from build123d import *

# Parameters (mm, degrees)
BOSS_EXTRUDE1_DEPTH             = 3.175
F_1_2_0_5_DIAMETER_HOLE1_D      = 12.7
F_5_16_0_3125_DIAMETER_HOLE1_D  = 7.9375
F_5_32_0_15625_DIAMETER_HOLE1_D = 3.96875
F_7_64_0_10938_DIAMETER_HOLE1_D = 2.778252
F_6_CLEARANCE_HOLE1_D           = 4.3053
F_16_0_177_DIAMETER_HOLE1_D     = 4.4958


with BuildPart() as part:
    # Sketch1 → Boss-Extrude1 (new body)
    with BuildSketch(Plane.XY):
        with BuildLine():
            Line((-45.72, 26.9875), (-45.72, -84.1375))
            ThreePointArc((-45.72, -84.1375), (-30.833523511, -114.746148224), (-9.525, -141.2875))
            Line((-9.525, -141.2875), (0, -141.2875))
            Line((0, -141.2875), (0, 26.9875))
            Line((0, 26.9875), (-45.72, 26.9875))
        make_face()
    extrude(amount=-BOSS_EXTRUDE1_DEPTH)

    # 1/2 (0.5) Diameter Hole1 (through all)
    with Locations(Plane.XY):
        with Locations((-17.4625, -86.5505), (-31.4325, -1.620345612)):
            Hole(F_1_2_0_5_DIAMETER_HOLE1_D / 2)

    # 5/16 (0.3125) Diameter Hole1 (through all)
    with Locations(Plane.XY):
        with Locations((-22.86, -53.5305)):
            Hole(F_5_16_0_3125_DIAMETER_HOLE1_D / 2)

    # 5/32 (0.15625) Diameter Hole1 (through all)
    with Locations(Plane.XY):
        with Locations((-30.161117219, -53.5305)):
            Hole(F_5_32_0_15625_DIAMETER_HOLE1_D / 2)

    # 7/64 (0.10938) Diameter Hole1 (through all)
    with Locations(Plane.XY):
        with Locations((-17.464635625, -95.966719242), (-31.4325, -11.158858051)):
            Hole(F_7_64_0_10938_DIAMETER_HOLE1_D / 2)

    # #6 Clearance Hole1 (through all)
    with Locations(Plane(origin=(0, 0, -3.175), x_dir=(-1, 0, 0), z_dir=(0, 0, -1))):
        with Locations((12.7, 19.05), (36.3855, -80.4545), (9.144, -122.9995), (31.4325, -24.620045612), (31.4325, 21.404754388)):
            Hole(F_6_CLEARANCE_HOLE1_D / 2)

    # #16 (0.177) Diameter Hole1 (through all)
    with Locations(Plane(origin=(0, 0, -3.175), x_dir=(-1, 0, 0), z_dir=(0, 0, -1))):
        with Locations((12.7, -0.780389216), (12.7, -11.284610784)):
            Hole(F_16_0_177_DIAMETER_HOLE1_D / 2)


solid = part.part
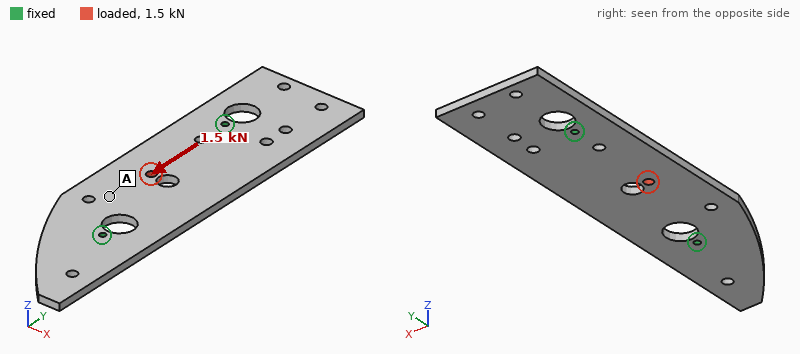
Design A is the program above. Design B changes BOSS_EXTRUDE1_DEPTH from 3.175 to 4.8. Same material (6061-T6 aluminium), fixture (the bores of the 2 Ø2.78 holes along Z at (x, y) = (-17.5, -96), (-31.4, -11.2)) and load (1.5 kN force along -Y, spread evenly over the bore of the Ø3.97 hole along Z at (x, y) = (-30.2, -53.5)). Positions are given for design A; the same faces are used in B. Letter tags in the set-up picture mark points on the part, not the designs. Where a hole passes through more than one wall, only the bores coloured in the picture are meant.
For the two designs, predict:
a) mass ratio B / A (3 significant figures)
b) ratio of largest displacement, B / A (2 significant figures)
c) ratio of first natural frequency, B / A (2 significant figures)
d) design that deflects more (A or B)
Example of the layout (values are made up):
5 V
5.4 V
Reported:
1.51
0.66
1.4
A
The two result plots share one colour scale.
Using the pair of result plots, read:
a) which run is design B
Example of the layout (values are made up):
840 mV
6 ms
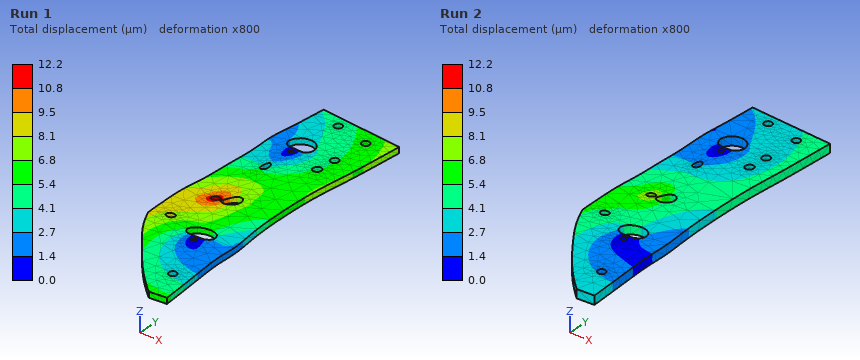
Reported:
Run 2
